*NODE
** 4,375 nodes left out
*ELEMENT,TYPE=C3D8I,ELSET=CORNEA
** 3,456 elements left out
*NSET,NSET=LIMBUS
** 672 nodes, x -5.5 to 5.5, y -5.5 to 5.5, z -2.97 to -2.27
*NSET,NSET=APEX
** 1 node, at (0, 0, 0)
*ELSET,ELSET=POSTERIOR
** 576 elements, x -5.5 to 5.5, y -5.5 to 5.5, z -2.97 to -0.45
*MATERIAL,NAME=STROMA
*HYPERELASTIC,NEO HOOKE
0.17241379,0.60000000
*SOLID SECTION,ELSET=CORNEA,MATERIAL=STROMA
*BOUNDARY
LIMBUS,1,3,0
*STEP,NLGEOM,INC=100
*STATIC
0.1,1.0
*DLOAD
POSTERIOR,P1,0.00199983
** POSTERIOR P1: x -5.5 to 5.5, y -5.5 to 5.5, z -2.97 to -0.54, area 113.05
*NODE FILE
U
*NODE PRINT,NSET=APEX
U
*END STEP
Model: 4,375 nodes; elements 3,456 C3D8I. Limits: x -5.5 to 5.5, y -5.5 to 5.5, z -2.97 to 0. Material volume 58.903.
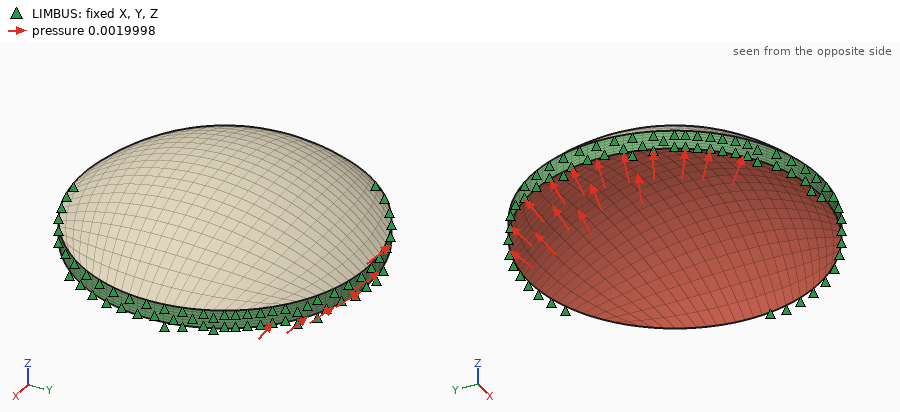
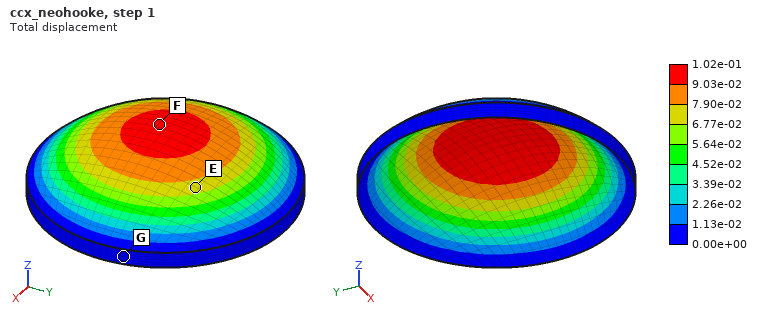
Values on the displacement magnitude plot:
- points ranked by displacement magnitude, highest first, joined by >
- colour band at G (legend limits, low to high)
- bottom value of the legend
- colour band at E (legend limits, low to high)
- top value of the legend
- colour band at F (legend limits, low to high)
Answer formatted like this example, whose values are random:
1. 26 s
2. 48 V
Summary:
1. F > E > G
2. 0.00e+00 to 1.13e-02
3. 0.00e+00
4. 6.77e-02 to 7.90e-02
5. 1.02e-01
6. 9.03e-02 to 1.02e-01
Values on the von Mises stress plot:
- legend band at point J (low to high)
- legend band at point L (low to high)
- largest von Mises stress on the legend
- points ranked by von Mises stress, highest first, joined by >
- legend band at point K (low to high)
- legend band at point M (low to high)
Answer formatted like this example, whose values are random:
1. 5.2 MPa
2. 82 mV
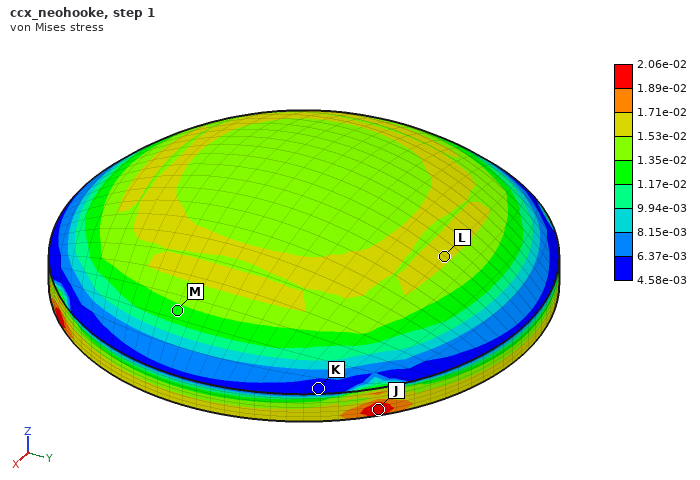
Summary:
1. 1.89e-02 to 2.06e-02
2. 1.53e-02 to 1.71e-02
3. 2.06e-02
4. J > L > M > K
5. 4.58e-03 to 6.37e-03
6. 1.17e-02 to 1.35e-02
